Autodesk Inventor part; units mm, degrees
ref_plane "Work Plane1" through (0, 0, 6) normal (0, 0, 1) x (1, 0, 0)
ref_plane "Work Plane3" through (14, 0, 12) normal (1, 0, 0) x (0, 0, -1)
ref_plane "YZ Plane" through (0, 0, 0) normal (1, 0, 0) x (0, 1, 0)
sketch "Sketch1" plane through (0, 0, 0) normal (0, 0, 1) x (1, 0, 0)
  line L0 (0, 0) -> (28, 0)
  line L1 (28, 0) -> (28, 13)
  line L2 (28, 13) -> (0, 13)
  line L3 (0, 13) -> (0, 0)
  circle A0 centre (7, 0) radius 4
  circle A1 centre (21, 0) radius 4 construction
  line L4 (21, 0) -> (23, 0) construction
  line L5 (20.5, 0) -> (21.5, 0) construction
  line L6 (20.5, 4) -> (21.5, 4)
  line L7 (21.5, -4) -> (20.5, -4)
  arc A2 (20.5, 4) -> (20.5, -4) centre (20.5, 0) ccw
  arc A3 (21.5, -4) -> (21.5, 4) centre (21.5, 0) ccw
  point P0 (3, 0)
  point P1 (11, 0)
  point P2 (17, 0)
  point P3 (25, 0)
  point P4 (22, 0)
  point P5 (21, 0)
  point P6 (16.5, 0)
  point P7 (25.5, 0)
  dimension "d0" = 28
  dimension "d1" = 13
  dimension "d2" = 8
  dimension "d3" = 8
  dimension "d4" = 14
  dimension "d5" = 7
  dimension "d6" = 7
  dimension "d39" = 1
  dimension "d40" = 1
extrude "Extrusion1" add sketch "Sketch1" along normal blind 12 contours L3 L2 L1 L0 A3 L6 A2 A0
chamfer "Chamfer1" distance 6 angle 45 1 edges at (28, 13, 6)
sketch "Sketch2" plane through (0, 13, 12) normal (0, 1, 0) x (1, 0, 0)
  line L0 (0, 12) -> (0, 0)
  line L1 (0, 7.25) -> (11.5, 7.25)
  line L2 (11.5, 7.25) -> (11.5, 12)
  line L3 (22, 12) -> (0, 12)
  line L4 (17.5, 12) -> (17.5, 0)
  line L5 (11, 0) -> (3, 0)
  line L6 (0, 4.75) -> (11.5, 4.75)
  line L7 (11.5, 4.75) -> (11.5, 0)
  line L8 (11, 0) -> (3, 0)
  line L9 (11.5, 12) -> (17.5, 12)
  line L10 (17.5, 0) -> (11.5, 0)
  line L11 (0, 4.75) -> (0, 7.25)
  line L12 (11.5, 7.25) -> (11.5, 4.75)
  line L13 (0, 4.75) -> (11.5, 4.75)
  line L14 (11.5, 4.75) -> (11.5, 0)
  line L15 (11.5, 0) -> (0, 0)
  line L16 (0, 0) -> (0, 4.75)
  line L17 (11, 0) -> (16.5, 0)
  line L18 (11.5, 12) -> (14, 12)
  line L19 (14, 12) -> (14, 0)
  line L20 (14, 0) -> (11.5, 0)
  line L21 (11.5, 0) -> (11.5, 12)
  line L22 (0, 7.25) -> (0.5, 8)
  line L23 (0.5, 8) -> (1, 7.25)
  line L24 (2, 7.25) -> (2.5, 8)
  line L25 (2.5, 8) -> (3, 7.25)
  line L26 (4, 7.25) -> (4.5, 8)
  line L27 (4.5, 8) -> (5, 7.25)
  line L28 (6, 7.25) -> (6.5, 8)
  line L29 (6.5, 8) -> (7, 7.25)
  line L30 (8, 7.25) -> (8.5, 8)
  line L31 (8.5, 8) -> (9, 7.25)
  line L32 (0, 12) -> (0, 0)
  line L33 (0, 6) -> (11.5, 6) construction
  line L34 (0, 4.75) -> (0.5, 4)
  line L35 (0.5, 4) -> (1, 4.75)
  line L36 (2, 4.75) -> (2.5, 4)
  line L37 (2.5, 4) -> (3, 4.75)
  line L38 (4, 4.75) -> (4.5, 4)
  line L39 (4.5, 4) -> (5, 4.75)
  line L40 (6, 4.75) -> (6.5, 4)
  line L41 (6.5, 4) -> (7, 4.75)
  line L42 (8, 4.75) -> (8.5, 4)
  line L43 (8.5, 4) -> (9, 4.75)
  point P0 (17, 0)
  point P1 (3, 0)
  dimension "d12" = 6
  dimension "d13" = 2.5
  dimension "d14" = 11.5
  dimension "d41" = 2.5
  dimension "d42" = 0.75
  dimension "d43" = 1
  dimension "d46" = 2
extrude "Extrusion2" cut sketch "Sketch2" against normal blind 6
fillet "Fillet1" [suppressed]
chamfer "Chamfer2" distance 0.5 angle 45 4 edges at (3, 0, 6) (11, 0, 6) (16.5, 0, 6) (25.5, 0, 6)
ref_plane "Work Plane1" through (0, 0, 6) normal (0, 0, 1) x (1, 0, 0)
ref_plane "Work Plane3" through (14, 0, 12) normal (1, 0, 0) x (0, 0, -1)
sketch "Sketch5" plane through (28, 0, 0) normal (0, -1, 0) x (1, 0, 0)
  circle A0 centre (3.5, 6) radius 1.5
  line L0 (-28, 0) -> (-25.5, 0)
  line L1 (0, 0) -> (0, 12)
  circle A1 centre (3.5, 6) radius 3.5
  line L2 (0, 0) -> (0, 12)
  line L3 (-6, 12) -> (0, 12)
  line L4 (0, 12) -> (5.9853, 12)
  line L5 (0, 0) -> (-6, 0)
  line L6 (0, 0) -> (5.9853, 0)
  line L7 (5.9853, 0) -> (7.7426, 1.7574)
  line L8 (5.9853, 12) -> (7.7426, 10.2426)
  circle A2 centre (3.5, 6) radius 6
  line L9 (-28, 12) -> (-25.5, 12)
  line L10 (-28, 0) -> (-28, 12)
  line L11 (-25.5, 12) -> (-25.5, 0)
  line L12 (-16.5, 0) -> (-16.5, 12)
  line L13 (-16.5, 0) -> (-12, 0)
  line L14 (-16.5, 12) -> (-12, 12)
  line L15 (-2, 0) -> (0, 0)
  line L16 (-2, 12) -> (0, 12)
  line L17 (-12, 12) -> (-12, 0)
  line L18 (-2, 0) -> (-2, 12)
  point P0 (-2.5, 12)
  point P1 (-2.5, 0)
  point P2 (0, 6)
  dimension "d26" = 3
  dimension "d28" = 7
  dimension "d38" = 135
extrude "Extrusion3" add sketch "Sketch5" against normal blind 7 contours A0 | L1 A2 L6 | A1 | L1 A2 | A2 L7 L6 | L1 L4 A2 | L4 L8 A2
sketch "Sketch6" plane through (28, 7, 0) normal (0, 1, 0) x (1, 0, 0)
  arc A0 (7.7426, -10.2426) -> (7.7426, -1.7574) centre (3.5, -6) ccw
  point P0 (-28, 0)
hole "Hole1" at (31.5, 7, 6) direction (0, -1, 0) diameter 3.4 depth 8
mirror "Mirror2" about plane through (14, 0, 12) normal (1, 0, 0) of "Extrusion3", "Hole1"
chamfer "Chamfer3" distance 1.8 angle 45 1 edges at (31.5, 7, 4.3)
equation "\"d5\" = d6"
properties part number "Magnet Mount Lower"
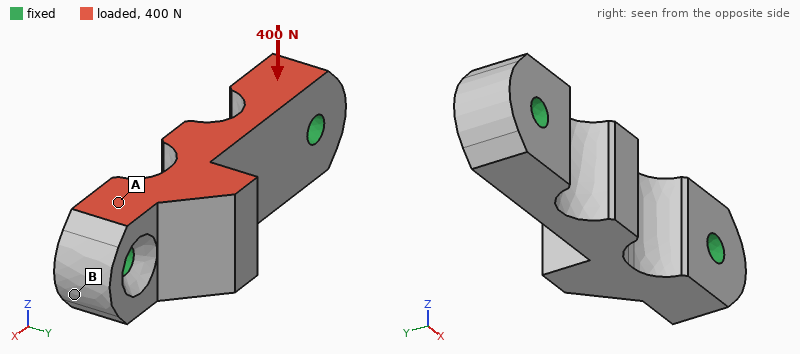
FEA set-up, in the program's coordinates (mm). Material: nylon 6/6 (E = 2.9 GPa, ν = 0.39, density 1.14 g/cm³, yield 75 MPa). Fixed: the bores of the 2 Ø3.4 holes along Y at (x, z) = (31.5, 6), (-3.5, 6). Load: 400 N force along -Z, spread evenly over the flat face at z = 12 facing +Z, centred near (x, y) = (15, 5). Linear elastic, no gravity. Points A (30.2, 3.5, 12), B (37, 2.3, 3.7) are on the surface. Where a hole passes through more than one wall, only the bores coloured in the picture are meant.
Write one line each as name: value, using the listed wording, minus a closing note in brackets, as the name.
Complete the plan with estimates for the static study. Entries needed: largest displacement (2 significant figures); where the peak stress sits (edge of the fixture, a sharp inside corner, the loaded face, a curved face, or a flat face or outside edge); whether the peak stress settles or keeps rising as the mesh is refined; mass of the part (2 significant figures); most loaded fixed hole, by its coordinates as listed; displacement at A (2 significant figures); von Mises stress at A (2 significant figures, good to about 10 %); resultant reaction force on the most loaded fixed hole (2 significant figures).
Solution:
largest displacement: 0.11 mm
where the peak stress sits: edge of the fixture
whether the peak stress settles or keeps rising as the mesh is refined: keeps rising
mass of the part: 4.0 g
most loaded fixed hole, by its coordinates as listed: (31.5, 6)
displacement at A: 0.026 mm
von Mises stress at A: 5.3 MPa
resultant reaction force on the most loaded fixed hole: 210 N
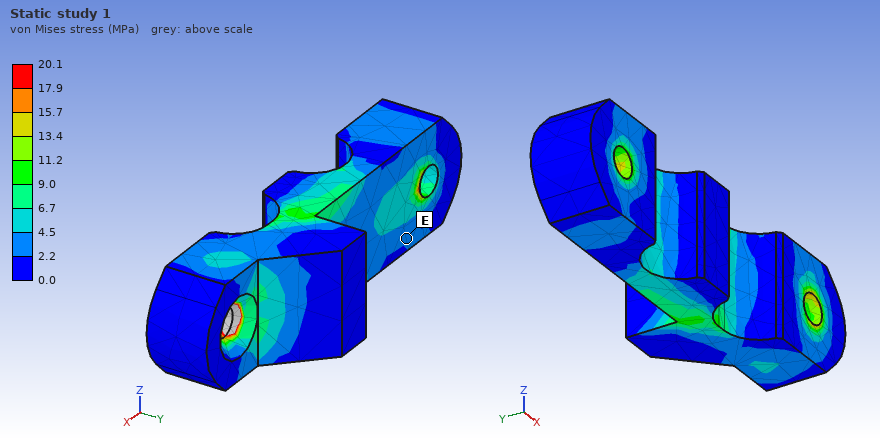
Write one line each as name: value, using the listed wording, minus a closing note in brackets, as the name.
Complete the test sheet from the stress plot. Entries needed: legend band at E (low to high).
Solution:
legend band at E: 2.2 to 4.5 MPa
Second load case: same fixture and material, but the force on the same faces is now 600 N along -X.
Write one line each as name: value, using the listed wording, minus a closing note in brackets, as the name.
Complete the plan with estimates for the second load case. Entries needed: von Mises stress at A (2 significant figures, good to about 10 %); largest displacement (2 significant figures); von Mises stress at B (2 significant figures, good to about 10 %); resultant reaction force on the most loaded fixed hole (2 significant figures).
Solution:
von Mises stress at A: 4.0 MPa
largest displacement: 81 µm
von Mises stress at B: 1.8 MPa
resultant reaction force on the most loaded fixed hole: 320 N
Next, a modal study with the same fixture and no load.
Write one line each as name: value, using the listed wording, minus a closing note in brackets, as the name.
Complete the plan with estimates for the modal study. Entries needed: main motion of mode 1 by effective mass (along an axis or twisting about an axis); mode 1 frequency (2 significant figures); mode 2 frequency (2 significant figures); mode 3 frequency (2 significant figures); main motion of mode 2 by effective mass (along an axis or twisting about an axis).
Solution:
main motion of mode 1 by effective mass: along Y
mode 1 frequency: 5800 Hz
mode 2 frequency: 6400 Hz
mode 3 frequency: 7900 Hz
main motion of mode 2 by effective mass: along Z
